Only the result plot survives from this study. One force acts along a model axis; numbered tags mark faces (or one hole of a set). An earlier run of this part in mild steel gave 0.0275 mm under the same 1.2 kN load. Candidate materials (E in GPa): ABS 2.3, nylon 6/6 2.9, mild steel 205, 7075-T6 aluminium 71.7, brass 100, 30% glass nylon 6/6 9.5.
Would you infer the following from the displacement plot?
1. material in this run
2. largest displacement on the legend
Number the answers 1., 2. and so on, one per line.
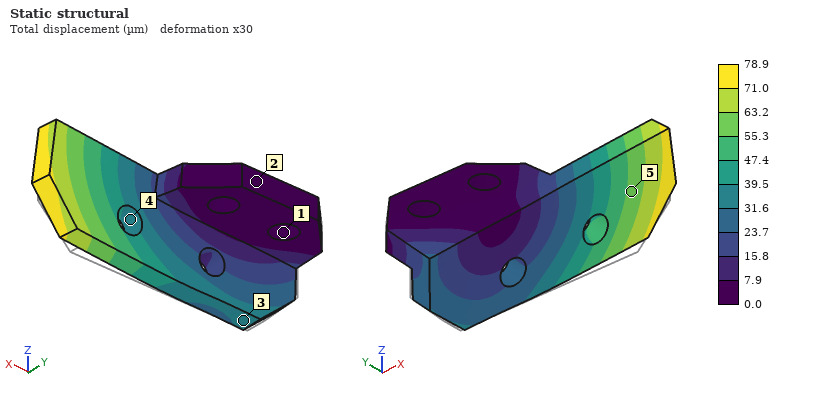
1. 7075-T6 aluminium
2. 78.9 µm
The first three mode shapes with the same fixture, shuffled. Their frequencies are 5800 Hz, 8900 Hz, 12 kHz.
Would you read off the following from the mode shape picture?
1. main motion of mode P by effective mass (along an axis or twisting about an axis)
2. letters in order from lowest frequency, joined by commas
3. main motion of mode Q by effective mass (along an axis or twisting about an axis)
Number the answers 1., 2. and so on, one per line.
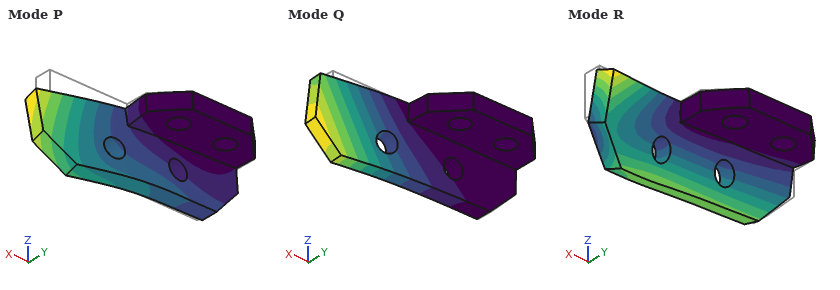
1. along Z
2. Q, P, R
3. along Y
